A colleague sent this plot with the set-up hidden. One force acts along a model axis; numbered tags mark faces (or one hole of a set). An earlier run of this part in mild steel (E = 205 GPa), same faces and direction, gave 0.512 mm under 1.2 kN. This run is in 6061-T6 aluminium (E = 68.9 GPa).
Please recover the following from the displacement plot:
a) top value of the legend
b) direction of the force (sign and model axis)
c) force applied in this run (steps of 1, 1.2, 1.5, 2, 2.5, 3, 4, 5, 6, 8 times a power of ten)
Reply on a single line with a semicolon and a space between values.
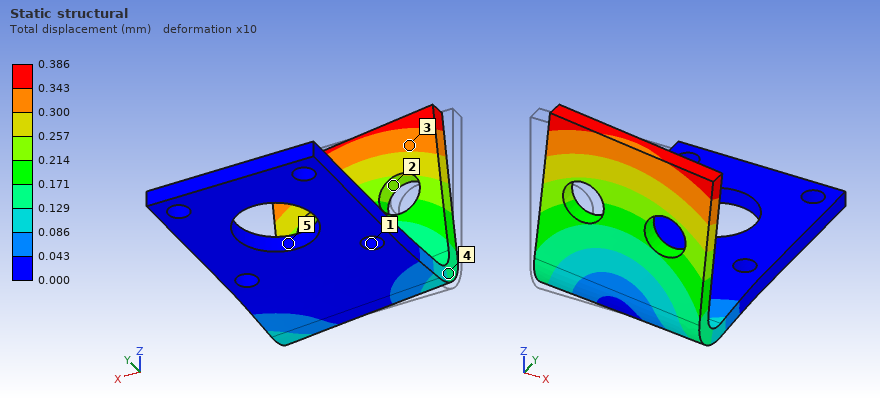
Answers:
0.386 mm; +X; 300 N
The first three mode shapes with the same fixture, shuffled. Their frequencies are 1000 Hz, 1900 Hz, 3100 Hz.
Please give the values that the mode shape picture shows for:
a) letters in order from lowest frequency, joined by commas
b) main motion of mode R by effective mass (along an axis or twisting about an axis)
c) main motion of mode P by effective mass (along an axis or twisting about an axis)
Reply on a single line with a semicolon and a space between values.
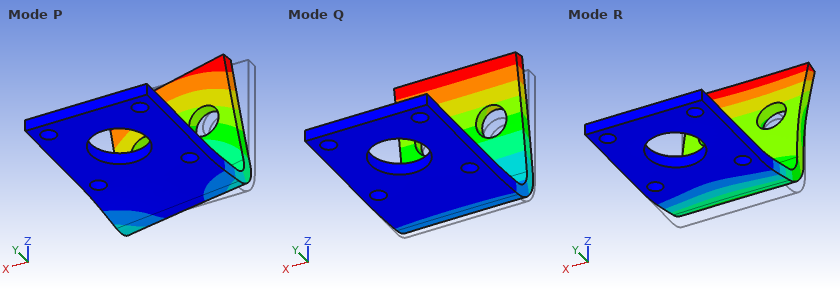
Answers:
Q, P, R; along Z; along X
